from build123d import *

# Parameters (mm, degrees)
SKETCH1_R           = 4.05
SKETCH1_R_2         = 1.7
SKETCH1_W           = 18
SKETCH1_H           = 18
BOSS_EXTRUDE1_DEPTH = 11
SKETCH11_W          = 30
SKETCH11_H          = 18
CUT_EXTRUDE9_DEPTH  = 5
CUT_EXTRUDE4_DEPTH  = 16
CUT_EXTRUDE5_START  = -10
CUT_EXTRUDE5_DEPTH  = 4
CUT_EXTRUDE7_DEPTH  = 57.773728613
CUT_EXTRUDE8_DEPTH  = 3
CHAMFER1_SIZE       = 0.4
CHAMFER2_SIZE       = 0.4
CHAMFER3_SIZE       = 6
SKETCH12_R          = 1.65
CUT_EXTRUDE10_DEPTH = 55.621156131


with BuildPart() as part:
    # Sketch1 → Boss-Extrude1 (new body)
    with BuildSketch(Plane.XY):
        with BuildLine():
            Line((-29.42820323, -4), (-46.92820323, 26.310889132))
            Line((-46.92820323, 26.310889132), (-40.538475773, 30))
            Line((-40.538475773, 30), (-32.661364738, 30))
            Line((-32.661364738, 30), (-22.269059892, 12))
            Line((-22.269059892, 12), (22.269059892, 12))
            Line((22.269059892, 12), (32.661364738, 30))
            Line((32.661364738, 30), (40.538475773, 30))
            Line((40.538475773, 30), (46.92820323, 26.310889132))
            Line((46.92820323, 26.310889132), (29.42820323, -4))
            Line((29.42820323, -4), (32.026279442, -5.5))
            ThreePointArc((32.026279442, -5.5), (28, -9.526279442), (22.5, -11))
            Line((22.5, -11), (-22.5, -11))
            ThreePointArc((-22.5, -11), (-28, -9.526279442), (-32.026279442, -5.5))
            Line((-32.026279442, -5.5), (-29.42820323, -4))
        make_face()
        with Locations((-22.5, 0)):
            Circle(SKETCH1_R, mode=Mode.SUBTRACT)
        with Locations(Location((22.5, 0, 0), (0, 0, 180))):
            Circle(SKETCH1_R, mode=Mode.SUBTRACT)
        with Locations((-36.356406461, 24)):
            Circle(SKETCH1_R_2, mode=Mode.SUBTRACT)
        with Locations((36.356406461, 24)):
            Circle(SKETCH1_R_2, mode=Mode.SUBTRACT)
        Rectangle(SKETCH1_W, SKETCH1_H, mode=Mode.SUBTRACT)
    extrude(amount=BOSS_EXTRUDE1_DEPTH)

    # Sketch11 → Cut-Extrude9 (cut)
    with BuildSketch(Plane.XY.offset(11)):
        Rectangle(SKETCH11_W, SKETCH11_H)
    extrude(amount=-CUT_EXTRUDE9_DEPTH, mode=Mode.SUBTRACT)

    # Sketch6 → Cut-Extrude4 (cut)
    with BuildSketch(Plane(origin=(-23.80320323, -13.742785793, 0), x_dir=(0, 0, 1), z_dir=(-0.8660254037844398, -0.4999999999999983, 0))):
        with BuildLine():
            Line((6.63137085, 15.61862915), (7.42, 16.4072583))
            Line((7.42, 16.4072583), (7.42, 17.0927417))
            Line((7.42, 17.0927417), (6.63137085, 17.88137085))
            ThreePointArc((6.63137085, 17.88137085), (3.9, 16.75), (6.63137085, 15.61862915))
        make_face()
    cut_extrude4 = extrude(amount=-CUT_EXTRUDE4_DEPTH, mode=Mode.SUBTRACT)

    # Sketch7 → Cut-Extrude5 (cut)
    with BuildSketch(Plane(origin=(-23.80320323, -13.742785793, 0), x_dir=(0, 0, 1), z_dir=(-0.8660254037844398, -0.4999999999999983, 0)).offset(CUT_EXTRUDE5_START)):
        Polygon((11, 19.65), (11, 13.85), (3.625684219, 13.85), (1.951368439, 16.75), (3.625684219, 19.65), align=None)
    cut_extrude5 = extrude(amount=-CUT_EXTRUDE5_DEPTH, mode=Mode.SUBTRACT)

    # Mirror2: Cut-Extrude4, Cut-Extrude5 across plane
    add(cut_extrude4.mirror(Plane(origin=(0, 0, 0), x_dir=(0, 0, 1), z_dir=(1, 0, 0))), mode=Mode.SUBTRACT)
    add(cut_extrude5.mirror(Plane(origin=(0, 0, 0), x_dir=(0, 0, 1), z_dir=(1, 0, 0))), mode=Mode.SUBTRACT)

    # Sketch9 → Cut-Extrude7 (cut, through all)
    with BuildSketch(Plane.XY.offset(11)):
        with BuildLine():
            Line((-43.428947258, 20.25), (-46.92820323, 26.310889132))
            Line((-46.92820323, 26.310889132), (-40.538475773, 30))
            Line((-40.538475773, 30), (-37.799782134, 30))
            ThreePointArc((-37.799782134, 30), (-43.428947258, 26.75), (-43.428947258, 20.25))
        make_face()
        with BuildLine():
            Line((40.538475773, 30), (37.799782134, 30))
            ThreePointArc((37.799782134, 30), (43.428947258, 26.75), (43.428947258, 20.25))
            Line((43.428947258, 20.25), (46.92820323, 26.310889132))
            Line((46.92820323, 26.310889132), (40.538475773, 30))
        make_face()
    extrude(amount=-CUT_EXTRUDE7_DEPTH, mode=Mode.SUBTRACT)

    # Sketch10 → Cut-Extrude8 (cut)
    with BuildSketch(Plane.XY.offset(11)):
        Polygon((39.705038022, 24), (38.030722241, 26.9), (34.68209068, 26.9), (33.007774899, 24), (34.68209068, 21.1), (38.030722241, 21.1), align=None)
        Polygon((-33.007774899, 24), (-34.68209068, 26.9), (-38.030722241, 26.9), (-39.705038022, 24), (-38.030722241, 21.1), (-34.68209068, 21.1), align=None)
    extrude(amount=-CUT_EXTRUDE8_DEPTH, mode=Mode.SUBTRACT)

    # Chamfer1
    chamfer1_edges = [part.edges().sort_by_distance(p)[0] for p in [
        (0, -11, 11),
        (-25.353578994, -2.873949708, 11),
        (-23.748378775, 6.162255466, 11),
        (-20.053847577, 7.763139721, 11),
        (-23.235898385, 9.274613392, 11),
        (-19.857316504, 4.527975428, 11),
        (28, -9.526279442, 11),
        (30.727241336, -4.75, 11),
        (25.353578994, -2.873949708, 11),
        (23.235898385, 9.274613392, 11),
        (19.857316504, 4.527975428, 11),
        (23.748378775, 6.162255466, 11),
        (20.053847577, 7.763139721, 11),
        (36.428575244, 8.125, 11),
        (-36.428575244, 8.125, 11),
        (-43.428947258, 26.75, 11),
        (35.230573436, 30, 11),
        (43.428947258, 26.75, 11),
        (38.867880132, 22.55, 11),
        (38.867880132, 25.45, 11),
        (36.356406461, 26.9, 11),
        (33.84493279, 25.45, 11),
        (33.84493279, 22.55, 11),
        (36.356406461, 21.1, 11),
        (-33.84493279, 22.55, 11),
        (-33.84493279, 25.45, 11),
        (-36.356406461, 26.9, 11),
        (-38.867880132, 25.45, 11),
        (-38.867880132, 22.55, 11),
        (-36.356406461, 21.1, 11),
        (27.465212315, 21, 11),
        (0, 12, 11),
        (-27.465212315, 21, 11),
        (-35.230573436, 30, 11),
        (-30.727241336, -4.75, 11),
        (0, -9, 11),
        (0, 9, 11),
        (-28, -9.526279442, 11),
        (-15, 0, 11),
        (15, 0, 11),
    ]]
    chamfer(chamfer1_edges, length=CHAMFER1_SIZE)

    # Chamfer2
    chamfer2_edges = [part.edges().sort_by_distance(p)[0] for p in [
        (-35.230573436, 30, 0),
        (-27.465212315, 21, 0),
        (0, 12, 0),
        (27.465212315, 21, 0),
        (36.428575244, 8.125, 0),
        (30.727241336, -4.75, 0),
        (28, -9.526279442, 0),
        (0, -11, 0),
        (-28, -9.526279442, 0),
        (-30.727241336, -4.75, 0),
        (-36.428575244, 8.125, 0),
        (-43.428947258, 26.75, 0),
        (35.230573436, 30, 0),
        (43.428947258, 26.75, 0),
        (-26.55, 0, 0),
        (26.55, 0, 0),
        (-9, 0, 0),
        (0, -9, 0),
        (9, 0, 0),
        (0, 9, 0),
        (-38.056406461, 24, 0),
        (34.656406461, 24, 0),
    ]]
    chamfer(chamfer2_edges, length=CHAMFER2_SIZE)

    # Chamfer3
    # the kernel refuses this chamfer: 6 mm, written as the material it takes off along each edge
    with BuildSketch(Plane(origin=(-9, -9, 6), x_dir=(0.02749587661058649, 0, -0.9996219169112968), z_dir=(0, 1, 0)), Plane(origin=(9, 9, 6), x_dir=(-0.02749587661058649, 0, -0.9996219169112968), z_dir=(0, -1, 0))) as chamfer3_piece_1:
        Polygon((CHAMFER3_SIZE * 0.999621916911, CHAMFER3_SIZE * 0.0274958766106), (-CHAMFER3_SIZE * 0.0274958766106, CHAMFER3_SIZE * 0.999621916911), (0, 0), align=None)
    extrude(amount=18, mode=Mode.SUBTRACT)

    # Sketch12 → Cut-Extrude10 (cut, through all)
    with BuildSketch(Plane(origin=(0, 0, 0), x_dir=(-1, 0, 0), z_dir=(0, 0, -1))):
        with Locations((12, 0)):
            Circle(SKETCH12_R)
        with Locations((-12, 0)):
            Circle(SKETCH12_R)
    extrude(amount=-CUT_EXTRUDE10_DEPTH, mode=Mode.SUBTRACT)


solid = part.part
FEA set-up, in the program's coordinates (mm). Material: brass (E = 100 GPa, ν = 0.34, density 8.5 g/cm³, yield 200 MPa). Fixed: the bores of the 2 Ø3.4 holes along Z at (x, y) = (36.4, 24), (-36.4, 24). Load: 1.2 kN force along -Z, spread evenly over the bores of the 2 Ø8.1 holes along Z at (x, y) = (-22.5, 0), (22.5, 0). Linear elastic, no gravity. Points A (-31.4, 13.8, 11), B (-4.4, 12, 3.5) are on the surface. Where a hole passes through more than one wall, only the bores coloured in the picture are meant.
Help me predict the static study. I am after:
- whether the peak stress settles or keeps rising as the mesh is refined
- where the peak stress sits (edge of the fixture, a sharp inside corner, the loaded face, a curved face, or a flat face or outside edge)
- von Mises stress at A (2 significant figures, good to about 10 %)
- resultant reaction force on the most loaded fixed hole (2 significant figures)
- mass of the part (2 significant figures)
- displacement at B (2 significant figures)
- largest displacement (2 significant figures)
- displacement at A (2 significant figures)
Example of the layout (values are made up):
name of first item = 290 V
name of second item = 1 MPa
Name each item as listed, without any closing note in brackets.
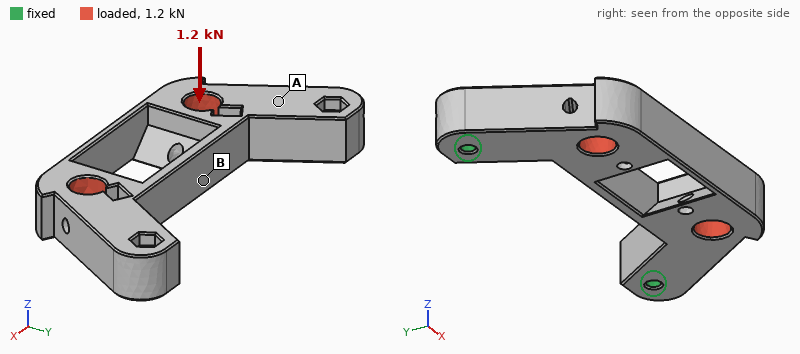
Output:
whether the peak stress settles or keeps rising as the mesh is refined = keeps rising
where the peak stress sits = edge of the fixture
von Mises stress at A = 30 MPa
resultant reaction force on the most loaded fixed hole = 600 N
mass of the part = 130 g
displacement at B = 30 µm
largest displacement = 81 µm
displacement at A = 17 µm
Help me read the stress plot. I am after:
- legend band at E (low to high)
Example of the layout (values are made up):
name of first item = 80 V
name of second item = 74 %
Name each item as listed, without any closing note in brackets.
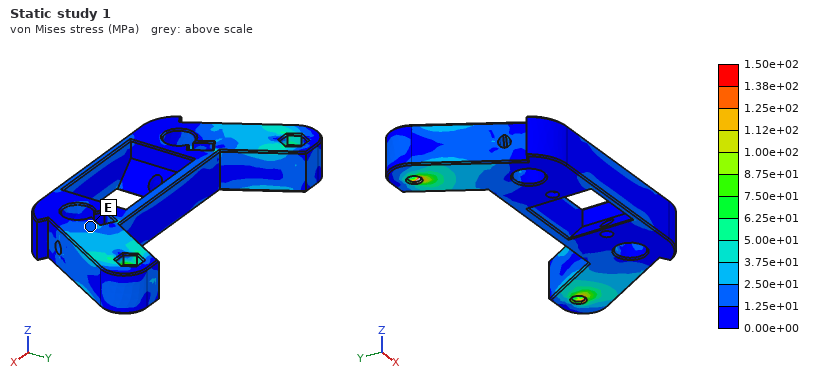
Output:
legend band at E = 1.25e+01 to 2.50e+01 MPa
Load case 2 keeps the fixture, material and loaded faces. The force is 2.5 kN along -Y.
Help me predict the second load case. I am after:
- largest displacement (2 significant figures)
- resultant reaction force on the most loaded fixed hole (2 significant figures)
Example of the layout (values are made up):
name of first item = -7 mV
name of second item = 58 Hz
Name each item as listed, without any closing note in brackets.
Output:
largest displacement = 12 µm
resultant reaction force on the most loaded fixed hole = 1.4 kN
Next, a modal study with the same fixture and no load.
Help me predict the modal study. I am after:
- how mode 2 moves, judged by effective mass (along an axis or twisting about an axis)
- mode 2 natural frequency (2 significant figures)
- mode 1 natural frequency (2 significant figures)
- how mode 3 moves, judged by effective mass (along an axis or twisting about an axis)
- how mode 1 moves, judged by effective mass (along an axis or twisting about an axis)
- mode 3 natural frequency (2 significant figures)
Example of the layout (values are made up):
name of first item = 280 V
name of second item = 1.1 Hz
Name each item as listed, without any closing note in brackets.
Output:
how mode 2 moves, judged by effective mass = along X
mode 2 natural frequency = 3200 Hz
mode 1 natural frequency = 2700 Hz
how mode 3 moves, judged by effective mass = twisting about Y
how mode 1 moves, judged by effective mass = along Z
mode 3 natural frequency = 4500 Hz
